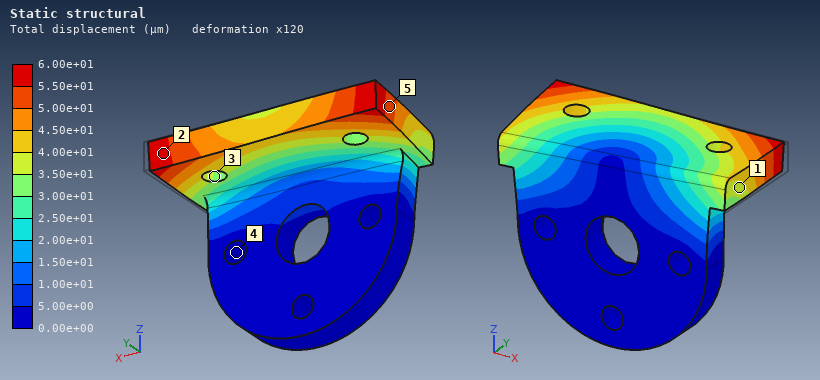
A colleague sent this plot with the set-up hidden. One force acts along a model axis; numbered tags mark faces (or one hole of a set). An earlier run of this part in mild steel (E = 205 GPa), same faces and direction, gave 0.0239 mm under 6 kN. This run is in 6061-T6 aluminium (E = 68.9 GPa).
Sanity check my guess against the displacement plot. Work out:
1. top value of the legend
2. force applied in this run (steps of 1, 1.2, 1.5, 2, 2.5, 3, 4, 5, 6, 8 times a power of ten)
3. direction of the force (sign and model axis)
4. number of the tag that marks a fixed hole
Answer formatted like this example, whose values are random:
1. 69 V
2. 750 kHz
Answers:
1. 6.00e+01 µm
2. 5 kN
3. -X
4. 4
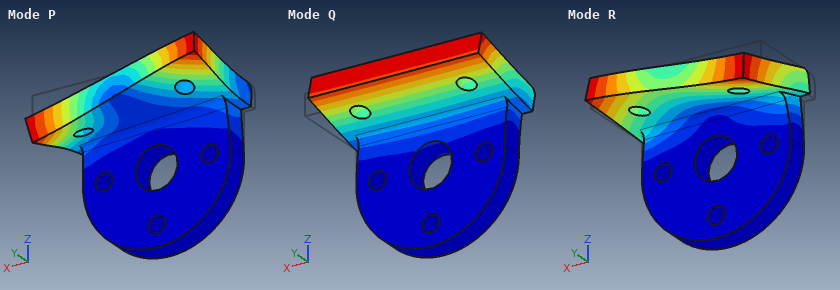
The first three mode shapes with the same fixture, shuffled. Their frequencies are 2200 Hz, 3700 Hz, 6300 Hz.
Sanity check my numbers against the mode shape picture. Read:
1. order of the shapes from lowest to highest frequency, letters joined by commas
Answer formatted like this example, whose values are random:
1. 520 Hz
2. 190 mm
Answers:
1. Q, R, P
